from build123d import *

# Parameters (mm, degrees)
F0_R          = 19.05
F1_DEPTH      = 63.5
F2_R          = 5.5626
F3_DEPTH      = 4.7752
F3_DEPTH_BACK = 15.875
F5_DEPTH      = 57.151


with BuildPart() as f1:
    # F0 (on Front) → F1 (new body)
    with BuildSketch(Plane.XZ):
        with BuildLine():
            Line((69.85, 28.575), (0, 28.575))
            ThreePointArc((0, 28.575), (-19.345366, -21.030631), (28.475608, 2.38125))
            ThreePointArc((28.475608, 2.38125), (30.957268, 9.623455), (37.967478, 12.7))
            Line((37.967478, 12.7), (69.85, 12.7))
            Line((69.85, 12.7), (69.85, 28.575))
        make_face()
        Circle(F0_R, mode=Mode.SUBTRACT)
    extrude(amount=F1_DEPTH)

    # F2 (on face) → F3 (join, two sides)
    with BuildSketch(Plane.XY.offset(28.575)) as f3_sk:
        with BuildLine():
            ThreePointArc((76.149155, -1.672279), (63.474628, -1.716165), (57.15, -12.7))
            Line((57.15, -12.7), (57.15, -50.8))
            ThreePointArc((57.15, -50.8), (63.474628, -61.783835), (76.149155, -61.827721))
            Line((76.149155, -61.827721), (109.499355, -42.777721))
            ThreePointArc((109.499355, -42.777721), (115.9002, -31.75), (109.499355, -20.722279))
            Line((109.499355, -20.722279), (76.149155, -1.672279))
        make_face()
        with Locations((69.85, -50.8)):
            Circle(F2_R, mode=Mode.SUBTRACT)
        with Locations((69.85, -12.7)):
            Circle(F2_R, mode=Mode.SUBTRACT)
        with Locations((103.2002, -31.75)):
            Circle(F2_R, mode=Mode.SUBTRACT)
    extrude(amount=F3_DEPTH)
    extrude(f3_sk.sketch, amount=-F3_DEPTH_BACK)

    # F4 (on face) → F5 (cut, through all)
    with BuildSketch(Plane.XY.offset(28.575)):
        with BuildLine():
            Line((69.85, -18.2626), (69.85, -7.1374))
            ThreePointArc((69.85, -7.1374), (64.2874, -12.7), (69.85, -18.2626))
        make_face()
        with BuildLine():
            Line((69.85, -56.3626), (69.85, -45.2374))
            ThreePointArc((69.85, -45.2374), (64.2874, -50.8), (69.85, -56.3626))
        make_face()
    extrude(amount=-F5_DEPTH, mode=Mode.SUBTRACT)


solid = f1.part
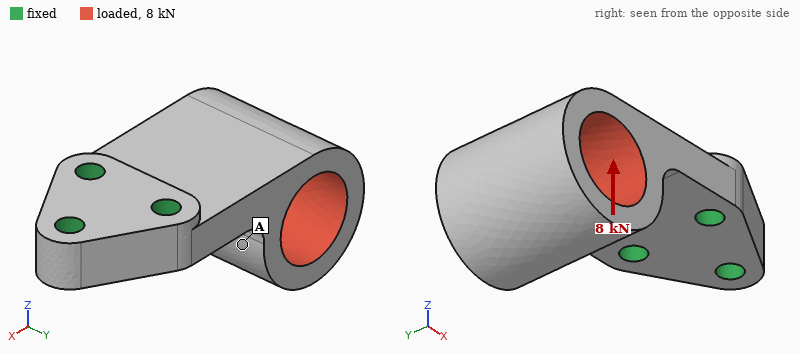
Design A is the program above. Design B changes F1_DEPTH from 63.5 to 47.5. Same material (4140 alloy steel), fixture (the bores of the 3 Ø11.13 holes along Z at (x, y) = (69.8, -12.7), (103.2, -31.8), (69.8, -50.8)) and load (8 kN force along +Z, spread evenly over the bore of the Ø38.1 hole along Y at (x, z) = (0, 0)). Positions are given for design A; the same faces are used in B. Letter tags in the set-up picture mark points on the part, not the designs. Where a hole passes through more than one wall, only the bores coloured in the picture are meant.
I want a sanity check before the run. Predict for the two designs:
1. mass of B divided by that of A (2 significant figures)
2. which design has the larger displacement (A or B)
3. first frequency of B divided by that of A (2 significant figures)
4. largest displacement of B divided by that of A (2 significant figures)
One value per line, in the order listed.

0.81
B
1.00
1.3
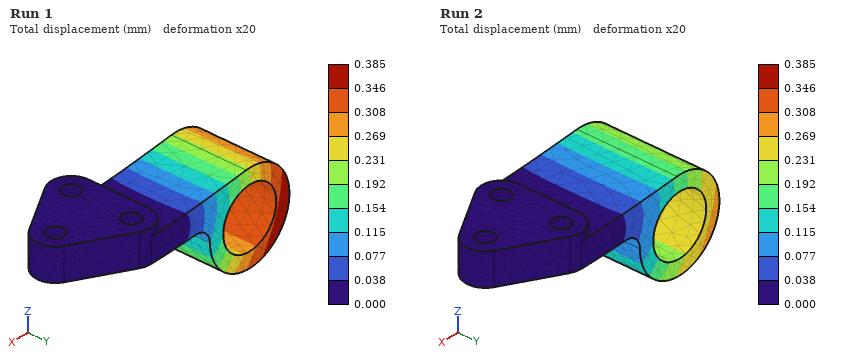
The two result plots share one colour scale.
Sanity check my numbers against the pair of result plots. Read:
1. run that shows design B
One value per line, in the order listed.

Run 1
